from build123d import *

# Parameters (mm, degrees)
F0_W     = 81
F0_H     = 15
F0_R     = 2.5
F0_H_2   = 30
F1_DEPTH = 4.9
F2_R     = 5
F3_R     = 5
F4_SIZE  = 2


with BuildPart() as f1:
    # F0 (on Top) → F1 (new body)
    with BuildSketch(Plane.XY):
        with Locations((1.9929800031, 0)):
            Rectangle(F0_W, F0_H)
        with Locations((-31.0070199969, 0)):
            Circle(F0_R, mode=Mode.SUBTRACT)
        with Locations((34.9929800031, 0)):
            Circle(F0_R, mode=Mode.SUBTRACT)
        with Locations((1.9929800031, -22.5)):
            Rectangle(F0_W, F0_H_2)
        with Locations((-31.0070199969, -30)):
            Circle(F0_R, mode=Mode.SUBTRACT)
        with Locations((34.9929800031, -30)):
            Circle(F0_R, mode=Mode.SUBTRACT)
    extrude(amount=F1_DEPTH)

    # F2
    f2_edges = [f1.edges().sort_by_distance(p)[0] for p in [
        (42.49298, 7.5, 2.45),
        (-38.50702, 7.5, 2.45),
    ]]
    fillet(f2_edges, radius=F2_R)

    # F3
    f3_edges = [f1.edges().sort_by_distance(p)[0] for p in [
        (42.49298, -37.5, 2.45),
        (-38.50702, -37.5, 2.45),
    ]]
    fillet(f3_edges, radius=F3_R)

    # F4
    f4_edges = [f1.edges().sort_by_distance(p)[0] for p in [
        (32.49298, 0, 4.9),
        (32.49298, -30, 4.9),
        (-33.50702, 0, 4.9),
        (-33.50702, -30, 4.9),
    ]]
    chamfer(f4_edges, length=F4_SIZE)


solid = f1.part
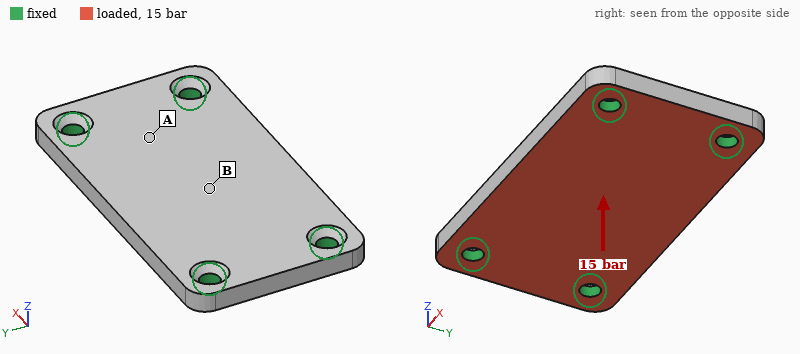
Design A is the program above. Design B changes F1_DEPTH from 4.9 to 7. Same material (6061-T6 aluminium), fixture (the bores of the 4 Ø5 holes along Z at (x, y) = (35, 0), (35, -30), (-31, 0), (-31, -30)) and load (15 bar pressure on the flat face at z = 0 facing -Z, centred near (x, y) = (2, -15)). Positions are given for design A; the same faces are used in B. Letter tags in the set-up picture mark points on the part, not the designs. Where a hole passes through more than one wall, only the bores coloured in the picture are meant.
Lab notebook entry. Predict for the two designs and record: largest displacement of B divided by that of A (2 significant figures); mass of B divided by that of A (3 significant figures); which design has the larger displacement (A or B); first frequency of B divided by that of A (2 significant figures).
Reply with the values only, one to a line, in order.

0.36
1.43
A
1.4
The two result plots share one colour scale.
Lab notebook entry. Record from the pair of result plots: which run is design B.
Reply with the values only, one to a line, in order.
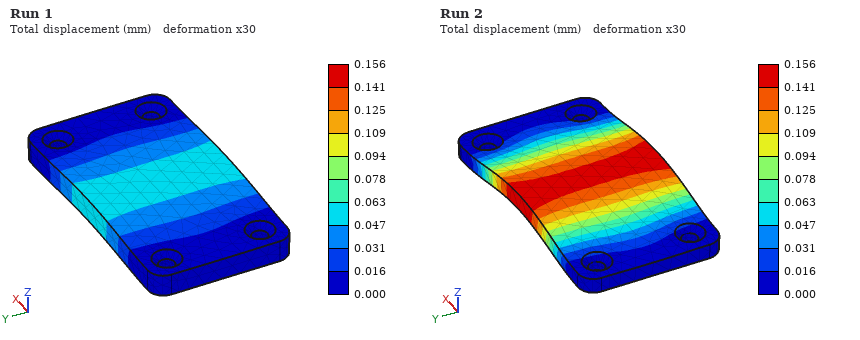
Run 1
